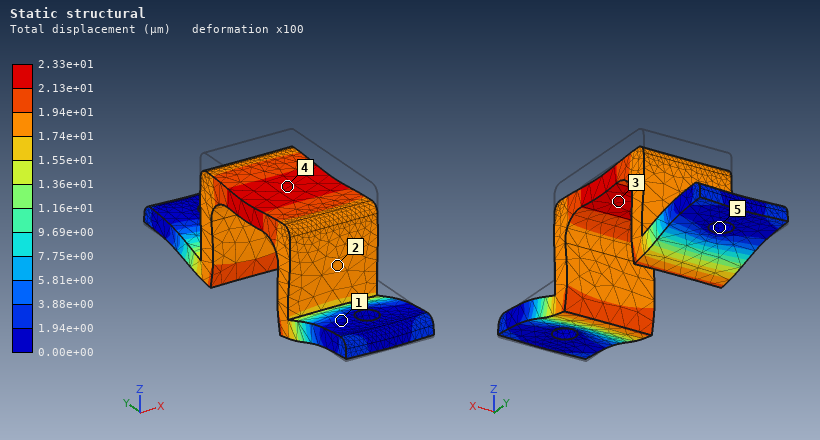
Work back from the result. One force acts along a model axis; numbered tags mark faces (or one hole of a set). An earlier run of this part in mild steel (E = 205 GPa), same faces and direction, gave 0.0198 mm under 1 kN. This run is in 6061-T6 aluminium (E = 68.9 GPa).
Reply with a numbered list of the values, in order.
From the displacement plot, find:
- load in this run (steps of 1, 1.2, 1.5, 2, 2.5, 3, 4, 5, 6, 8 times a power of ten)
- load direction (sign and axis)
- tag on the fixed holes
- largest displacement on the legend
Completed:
1. 400 N
2. -Z
3. 5
4. 2.33e+01 µm
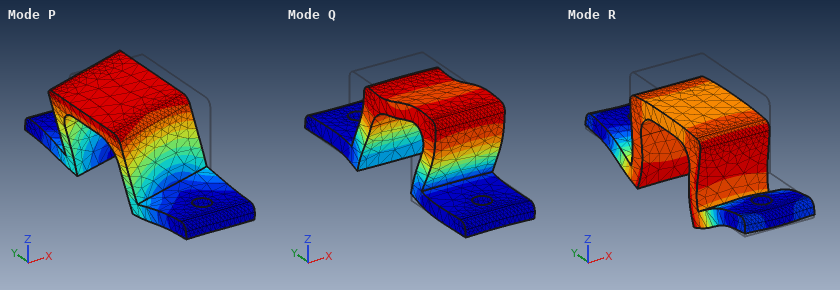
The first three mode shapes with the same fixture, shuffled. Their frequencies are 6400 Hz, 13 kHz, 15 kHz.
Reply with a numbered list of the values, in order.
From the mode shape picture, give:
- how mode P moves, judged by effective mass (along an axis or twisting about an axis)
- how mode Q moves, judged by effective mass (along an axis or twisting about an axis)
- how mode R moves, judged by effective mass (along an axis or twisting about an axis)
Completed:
1. along X
2. along Y
3. along Z
